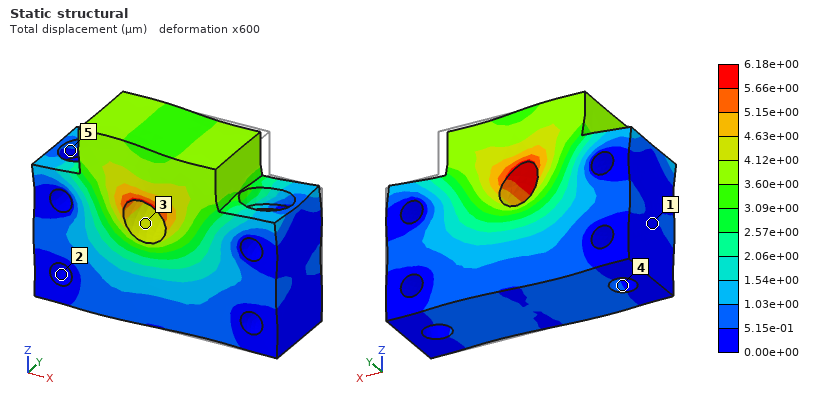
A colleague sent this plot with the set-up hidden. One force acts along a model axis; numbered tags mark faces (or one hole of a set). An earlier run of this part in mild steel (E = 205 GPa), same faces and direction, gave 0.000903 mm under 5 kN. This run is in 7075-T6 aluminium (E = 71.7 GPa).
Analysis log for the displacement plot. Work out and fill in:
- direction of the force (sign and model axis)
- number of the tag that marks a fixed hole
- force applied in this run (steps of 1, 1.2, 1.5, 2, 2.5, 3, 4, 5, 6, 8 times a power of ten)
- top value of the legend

-X
2
12 kN
6.18e+00 µm
